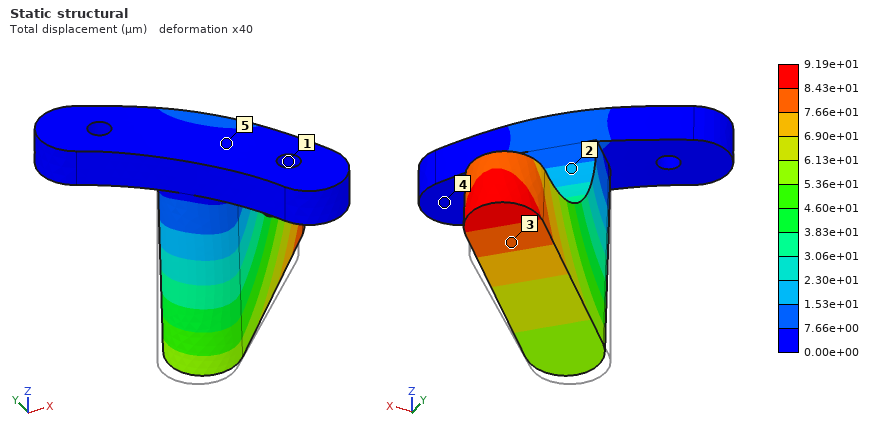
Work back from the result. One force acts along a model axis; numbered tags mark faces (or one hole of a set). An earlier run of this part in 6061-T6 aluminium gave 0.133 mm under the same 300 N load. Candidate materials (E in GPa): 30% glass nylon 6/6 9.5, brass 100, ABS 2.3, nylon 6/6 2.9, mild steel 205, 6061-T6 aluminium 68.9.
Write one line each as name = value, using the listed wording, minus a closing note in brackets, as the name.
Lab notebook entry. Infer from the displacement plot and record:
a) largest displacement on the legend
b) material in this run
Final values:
largest displacement on the legend = 9.19e+01 µm
material in this run = brass
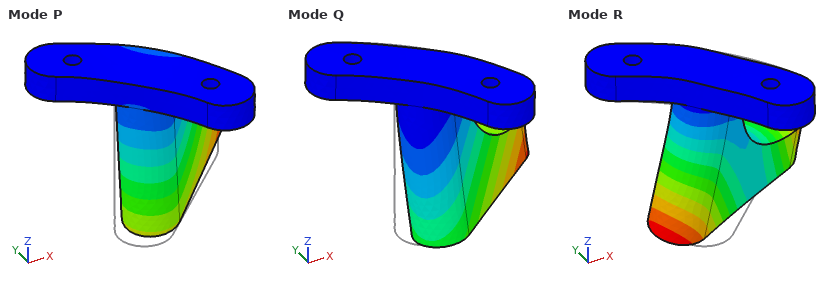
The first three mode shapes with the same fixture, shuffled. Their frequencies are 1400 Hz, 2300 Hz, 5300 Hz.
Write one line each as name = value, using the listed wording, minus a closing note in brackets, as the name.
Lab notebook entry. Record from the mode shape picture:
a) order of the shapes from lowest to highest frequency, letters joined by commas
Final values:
order of the shapes from lowest to highest frequency, letters joined by commas = P, Q, R
